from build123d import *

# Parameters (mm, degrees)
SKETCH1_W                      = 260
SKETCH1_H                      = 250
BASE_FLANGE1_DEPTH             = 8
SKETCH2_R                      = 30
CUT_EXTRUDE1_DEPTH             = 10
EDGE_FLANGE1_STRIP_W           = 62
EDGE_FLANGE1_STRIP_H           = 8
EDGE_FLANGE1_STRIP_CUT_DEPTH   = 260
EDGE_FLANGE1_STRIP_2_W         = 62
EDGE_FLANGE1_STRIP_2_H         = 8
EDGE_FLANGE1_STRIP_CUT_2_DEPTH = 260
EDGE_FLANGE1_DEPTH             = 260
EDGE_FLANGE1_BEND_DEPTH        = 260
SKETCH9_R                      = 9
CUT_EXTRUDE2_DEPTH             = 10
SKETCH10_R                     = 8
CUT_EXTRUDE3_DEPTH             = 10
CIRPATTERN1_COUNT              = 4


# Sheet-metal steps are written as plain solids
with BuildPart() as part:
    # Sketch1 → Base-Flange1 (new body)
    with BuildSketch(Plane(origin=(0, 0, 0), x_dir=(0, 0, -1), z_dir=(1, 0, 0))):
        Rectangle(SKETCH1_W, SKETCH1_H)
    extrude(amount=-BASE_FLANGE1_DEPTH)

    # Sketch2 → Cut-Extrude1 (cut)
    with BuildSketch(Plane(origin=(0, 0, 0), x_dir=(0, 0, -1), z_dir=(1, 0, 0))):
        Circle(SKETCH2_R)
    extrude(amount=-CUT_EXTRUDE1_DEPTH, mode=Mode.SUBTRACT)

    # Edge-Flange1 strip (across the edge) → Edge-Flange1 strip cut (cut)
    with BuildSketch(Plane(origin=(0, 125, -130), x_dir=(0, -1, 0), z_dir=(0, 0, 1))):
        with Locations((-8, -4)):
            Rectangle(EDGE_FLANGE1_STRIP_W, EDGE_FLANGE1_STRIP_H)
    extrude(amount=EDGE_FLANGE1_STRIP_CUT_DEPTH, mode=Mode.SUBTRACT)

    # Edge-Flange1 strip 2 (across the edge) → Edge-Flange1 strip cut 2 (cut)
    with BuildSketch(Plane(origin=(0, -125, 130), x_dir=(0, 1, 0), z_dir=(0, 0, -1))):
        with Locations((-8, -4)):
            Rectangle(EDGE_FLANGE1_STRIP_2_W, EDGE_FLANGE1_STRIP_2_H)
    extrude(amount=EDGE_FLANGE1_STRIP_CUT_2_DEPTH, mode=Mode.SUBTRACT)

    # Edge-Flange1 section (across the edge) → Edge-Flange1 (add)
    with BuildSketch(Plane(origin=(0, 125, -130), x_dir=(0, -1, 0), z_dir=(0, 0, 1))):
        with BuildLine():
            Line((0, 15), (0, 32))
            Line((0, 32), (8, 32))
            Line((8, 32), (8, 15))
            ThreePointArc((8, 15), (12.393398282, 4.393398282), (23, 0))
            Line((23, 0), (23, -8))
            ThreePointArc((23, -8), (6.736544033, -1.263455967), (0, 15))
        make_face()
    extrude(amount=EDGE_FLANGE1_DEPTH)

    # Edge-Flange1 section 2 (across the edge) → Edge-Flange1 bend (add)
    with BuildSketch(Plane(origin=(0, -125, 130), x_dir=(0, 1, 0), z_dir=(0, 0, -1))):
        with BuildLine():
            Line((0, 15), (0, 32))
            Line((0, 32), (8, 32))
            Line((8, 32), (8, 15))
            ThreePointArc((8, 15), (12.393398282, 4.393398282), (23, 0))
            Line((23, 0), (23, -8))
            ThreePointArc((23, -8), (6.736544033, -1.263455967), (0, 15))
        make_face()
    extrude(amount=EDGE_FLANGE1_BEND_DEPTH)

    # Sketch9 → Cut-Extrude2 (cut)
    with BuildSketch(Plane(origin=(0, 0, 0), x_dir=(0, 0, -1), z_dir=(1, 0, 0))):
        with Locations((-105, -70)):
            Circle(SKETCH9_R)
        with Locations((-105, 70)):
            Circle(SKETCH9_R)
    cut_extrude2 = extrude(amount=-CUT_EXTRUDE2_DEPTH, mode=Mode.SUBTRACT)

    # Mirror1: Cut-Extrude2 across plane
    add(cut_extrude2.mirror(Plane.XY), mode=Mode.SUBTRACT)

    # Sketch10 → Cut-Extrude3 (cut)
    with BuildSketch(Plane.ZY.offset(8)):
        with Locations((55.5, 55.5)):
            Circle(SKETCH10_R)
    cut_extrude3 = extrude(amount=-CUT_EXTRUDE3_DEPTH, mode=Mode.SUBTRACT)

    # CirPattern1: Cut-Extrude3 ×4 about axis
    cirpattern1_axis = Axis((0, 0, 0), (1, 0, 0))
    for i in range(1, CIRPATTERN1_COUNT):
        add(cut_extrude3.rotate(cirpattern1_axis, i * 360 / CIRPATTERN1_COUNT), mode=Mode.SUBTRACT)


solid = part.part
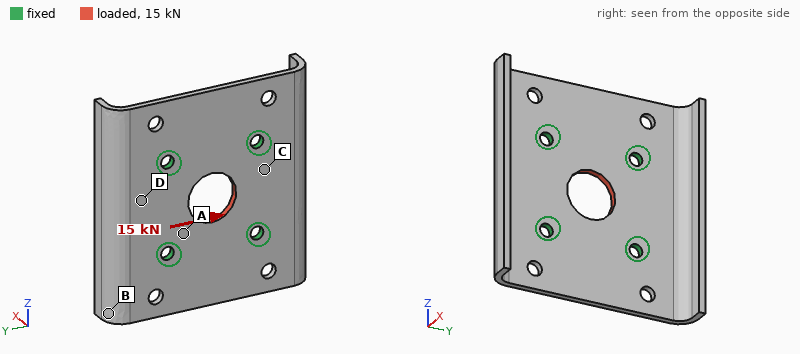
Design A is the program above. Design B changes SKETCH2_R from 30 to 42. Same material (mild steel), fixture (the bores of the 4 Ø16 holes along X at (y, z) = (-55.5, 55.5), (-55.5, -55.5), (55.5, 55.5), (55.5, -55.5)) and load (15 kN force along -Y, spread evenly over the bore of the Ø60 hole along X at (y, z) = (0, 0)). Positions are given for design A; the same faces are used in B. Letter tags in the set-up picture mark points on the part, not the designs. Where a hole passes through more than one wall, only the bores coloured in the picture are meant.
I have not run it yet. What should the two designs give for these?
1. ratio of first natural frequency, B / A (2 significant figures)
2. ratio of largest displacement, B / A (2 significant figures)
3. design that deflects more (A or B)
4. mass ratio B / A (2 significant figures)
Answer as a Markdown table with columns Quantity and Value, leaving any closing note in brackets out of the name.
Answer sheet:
| Quantity | Value |
|---|---|
| ratio of first natural frequency, B / A | 0.99 |
| ratio of largest displacement, B / A | 0.87 |
| design that deflects more | A |
| mass ratio B / A | 0.96 |
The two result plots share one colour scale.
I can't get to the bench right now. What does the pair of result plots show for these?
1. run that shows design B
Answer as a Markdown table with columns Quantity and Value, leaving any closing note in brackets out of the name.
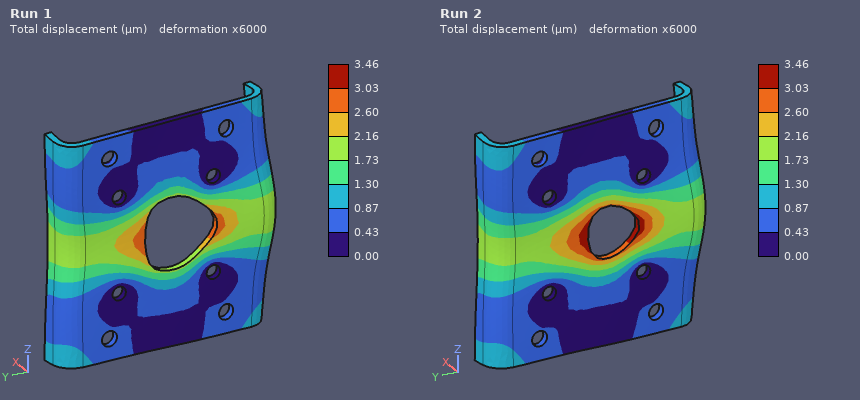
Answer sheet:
| Quantity | Value |
|---|---|
| run that shows design B | Run 1 |
